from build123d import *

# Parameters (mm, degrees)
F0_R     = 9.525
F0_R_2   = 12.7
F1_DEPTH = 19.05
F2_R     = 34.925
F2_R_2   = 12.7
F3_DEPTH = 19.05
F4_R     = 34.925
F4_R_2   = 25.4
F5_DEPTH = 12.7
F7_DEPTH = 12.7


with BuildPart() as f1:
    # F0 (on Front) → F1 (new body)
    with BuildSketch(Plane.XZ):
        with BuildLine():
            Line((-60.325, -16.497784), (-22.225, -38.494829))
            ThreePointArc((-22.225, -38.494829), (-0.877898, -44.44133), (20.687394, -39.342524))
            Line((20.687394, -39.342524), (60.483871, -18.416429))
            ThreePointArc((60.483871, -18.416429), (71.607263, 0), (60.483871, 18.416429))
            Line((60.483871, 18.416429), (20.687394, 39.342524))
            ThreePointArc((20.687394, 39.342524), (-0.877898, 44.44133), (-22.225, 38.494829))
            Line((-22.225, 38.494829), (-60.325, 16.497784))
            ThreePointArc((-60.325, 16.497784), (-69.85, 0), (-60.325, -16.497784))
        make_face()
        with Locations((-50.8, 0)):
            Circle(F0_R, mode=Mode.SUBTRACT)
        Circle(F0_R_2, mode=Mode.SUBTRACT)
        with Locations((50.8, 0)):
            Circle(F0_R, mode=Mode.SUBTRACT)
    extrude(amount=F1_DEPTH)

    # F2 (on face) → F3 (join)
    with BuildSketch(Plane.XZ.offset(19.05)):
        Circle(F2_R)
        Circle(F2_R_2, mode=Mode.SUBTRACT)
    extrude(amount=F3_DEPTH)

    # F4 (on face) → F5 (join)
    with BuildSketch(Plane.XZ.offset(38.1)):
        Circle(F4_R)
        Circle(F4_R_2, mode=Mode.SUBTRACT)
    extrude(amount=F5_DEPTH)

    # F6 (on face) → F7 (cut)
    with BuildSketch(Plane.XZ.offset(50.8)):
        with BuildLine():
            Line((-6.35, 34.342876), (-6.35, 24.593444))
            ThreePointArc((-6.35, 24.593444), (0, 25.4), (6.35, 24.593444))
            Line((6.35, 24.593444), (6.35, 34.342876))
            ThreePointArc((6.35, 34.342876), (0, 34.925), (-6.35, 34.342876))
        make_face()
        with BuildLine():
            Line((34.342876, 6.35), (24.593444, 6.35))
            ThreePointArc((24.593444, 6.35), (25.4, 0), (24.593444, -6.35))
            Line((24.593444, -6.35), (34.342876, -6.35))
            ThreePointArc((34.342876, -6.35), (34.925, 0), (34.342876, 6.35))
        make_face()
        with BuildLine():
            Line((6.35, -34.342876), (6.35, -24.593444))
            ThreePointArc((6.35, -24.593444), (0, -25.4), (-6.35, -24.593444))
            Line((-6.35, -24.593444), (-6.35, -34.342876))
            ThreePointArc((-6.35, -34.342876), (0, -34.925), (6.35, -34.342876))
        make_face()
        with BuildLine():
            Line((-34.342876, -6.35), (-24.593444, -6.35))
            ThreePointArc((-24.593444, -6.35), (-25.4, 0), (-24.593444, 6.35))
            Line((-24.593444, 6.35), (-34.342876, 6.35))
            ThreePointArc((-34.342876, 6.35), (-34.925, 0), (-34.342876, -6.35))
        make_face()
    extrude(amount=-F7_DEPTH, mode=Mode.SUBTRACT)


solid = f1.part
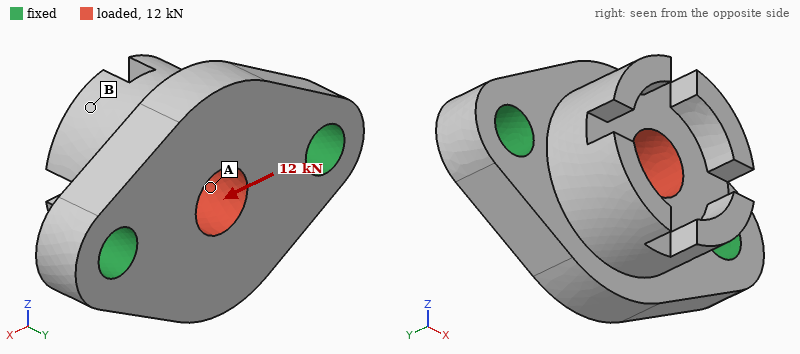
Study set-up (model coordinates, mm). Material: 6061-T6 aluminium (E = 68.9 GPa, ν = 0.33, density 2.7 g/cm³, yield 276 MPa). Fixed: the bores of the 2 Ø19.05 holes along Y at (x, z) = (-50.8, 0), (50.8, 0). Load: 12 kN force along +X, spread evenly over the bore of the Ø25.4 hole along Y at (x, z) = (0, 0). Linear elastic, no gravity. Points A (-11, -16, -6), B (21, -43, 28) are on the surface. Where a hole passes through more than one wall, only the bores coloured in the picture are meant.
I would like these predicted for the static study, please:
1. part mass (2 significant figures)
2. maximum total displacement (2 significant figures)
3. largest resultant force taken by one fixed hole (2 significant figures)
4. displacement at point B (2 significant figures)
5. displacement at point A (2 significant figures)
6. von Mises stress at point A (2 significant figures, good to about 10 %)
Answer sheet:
600 g
5.4 µm
6.2 kN
4.4 µm
3.5 µm
5.5 MPa
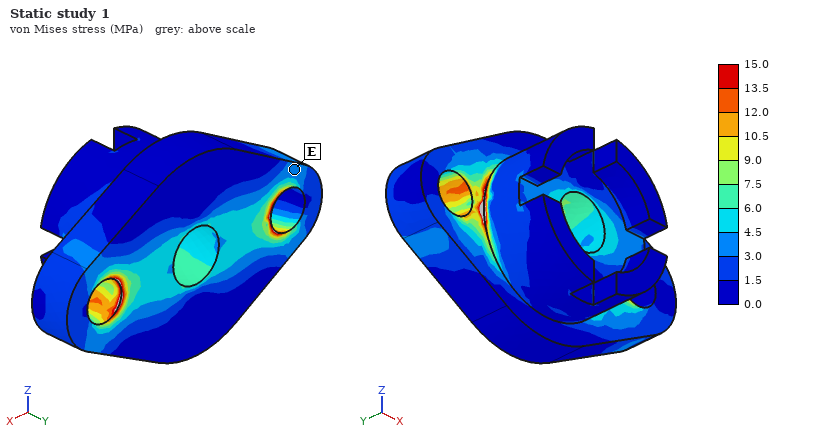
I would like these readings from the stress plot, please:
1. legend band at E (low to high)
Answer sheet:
3.0 to 4.5 MPa
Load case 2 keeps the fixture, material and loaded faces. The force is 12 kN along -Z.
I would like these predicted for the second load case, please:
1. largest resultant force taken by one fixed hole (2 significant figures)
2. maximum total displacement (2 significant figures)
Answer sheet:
6.0 kN
25 µm
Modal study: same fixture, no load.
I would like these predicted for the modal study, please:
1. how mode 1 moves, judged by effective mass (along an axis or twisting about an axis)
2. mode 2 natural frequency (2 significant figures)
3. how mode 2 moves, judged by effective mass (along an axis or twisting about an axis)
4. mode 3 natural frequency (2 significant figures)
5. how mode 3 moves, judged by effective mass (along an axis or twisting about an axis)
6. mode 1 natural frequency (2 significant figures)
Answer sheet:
along Z
7200 Hz
along Y
11 kHz
along Z
4600 Hz
